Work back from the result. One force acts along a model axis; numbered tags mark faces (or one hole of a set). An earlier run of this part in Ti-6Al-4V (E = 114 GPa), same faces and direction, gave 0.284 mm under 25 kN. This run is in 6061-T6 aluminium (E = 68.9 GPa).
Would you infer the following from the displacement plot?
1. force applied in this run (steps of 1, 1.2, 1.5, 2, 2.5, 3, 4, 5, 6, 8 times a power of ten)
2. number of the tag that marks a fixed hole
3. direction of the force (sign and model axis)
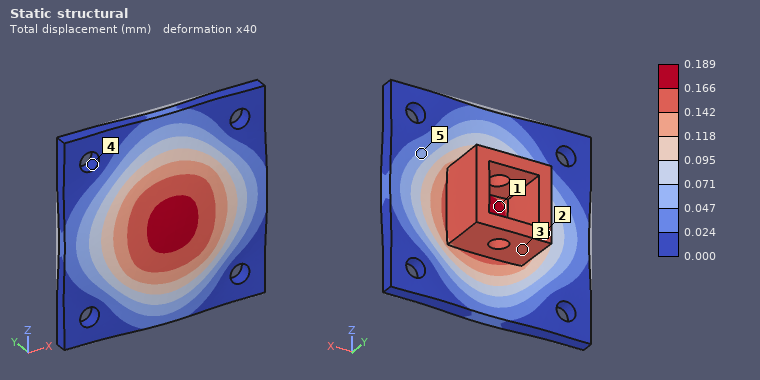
10 kN
4
-Y
